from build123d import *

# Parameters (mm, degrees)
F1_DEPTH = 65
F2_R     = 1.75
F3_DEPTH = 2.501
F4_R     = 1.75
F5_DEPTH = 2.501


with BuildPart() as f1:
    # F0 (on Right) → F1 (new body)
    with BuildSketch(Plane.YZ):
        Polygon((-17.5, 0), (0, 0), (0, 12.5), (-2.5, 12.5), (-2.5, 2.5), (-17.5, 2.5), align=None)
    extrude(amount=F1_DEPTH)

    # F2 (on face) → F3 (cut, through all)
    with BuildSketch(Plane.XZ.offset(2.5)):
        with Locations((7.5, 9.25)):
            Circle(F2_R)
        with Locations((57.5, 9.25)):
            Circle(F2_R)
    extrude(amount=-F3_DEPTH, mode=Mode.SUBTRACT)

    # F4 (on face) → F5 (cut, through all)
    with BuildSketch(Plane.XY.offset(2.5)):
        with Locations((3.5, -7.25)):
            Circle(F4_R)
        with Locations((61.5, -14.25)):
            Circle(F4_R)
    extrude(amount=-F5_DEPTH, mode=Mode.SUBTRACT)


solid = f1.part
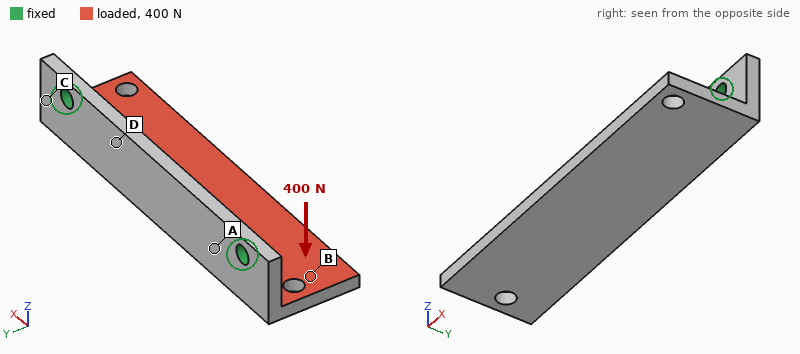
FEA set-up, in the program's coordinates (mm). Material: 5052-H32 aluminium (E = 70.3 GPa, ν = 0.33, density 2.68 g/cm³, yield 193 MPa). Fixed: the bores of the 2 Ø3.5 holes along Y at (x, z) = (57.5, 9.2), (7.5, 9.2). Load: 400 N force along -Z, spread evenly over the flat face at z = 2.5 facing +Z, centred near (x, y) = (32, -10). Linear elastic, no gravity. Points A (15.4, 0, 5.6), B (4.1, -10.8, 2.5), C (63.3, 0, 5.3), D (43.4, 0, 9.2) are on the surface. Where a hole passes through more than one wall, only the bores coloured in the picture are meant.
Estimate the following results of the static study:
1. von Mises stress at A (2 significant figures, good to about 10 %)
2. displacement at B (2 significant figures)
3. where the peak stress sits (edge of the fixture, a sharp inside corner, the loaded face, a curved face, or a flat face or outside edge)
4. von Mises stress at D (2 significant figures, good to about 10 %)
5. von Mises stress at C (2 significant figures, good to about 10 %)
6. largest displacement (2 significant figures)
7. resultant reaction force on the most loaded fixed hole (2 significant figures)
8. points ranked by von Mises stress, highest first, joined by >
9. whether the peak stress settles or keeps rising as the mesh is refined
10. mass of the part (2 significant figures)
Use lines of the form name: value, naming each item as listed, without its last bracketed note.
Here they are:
von Mises stress at A: 50 MPa
displacement at B: 0.082 mm
where the peak stress sits: edge of the fixture
von Mises stress at D: 33 MPa
von Mises stress at C: 66 MPa
largest displacement: 0.18 mm
resultant reaction force on the most loaded fixed hole: 220 N
points ranked by von Mises stress, highest first, joined by >: C > A > D > B
whether the peak stress settles or keeps rising as the mesh is refined: keeps rising
mass of the part: 12 g
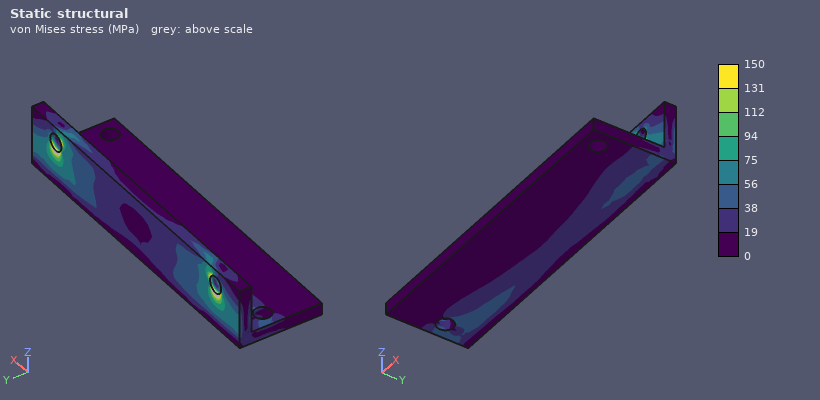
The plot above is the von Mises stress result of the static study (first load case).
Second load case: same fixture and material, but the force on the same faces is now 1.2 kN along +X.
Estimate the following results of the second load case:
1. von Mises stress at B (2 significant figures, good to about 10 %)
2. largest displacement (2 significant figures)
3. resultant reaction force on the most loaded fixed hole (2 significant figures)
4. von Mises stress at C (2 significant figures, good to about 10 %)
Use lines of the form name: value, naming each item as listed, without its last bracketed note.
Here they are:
von Mises stress at B: 16 MPa
largest displacement: 69 µm
resultant reaction force on the most loaded fixed hole: 650 N
von Mises stress at C: 34 MPa
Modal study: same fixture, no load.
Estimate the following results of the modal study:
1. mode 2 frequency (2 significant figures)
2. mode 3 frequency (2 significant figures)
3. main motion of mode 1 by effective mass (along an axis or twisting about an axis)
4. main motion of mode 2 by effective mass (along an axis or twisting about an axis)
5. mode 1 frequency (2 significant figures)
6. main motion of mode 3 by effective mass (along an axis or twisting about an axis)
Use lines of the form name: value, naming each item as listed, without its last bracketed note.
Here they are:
mode 2 frequency: 5900 Hz
mode 3 frequency: 8200 Hz
main motion of mode 1 by effective mass: along Z
main motion of mode 2 by effective mass: twisting about Y
mode 1 frequency: 3500 Hz
main motion of mode 3 by effective mass: along Y
